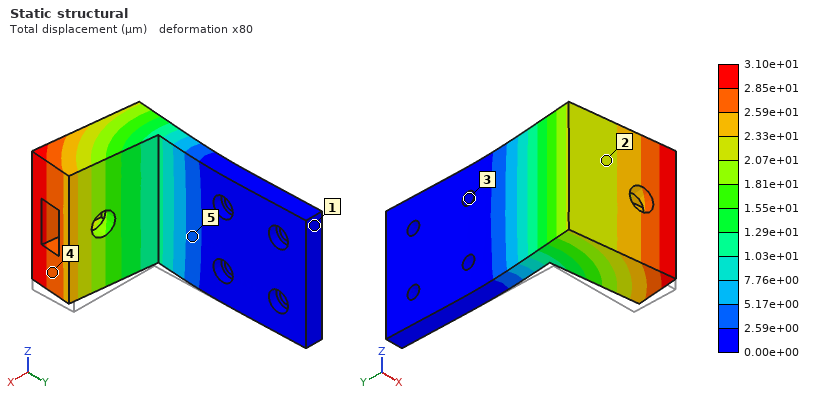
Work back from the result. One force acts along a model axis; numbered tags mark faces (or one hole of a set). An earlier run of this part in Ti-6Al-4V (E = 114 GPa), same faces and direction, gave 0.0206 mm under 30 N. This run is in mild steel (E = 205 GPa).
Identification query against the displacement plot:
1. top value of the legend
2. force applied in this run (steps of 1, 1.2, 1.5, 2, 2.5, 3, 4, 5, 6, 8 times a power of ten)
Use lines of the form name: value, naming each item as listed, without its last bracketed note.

top value of the legend: 3.10e+01 µm
force applied in this run: 80 N
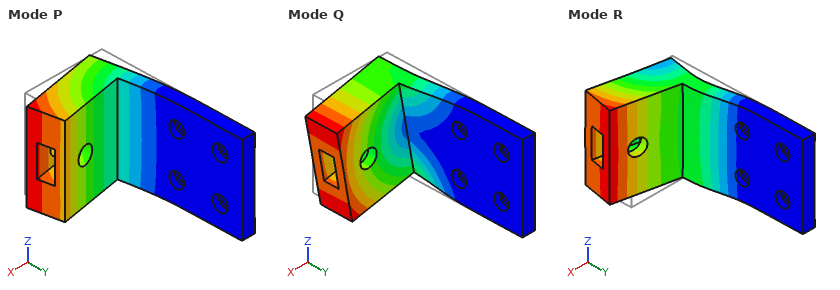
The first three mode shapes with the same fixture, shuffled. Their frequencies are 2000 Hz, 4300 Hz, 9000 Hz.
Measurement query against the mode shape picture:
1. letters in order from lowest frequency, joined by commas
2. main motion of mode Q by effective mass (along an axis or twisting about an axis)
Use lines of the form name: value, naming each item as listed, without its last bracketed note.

letters in order from lowest frequency, joined by commas: P, Q, R
main motion of mode Q by effective mass: along Z
